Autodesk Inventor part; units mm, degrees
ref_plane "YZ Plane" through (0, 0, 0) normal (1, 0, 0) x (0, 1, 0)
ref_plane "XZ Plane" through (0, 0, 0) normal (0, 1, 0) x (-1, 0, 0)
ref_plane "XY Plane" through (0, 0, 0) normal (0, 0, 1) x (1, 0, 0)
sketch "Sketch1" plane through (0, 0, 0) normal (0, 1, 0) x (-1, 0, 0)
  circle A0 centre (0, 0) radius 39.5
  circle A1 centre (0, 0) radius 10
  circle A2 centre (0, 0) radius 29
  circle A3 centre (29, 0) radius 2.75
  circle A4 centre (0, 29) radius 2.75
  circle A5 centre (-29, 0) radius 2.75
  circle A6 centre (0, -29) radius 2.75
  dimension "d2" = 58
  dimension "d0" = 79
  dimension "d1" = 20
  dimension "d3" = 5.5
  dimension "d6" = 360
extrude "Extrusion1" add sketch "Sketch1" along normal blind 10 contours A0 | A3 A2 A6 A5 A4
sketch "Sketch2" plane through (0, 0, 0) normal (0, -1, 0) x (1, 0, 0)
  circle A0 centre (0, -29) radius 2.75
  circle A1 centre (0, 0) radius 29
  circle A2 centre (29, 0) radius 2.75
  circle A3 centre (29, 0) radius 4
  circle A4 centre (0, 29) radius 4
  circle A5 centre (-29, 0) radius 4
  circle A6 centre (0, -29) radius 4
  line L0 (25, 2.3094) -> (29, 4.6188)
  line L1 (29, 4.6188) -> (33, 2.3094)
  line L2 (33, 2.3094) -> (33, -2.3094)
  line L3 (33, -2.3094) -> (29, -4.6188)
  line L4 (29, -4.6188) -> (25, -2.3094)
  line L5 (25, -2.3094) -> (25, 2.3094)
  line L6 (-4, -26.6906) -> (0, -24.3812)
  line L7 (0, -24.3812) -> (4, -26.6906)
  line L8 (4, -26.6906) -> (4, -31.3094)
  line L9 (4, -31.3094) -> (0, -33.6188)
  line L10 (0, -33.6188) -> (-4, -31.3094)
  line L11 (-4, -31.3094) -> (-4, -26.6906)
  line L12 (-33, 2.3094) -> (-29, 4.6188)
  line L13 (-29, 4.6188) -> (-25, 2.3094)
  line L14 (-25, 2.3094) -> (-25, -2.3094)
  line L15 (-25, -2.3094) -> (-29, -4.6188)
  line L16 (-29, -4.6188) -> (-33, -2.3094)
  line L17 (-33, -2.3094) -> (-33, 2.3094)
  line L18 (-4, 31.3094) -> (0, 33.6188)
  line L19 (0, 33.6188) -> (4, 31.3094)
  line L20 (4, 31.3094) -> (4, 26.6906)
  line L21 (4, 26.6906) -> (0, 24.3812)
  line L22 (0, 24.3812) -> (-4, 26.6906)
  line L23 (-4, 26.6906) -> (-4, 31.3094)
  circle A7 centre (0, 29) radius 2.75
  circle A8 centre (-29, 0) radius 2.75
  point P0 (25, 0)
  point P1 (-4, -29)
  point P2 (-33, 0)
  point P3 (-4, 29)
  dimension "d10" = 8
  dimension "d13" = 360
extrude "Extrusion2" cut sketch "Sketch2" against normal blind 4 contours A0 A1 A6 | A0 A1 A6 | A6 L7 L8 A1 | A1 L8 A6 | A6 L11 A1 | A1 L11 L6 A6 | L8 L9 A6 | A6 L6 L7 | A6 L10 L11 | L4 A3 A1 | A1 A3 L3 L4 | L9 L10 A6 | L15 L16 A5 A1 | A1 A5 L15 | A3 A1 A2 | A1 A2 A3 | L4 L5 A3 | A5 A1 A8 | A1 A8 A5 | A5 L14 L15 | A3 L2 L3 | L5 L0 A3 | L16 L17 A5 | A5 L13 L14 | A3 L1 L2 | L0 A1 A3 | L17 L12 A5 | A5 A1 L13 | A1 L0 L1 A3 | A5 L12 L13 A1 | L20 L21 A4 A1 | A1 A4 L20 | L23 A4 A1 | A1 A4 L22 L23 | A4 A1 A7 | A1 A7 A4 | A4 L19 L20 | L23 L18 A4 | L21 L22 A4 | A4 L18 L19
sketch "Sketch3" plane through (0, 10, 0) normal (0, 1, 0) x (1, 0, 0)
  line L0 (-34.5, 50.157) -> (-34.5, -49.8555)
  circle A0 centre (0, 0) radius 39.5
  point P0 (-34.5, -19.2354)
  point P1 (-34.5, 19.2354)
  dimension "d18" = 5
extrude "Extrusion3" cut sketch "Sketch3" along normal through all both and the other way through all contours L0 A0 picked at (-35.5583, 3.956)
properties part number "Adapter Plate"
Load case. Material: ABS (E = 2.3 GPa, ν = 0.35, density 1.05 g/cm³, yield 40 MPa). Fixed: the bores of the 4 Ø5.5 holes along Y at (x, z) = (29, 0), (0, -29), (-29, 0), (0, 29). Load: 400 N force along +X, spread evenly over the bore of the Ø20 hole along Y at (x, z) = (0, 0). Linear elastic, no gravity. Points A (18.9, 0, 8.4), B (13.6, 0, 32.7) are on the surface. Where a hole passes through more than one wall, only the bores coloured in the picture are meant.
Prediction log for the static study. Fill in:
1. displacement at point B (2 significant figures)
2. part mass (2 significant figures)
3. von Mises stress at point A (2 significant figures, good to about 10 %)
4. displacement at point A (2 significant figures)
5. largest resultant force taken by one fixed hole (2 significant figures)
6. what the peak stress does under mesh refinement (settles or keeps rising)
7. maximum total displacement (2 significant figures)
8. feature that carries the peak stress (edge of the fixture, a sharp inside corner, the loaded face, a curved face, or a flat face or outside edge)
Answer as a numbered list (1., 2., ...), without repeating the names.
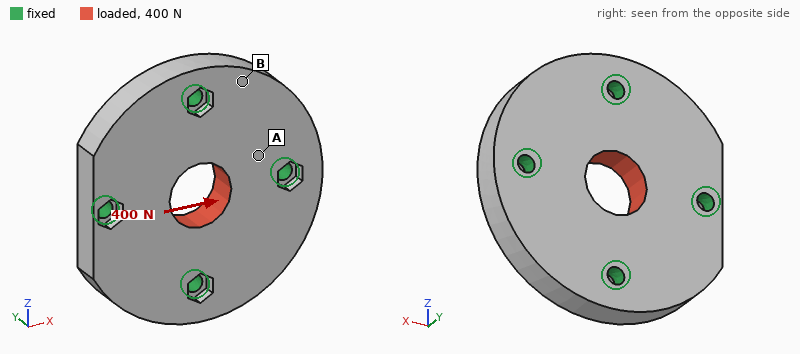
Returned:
1. 3.3 µm
2. 45 g
3. 0.48 MPa
4. 5.5 µm
5. 120 N
6. keeps rising
7. 8.7 µm
8. edge of the fixture
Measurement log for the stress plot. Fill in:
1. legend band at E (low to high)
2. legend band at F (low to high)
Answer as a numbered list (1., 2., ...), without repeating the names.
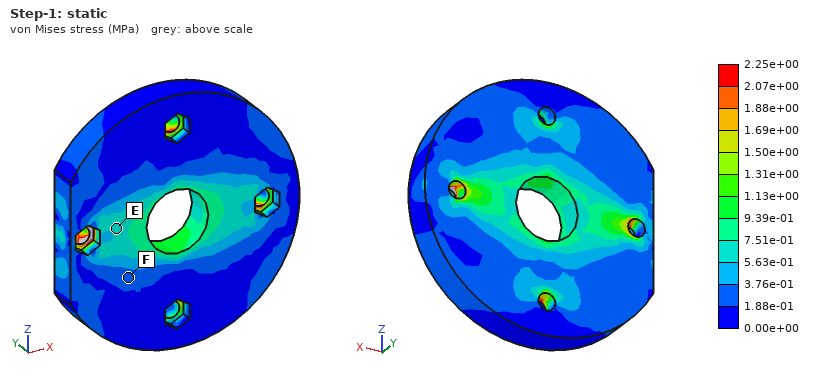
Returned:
1. 5.63e-01 to 7.51e-01 MPa
2. 1.88e-01 to 3.76e-01 MPa
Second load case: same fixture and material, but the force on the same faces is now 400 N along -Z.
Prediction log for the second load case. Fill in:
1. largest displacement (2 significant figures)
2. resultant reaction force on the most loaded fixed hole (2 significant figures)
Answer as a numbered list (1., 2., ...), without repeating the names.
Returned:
1. 8.7 µm
2. 120 N
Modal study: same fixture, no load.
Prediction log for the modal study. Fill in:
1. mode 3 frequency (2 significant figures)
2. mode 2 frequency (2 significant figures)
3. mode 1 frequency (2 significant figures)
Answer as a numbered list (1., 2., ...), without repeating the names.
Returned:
1. 4100 Hz
2. 3900 Hz
3. 3500 Hz
